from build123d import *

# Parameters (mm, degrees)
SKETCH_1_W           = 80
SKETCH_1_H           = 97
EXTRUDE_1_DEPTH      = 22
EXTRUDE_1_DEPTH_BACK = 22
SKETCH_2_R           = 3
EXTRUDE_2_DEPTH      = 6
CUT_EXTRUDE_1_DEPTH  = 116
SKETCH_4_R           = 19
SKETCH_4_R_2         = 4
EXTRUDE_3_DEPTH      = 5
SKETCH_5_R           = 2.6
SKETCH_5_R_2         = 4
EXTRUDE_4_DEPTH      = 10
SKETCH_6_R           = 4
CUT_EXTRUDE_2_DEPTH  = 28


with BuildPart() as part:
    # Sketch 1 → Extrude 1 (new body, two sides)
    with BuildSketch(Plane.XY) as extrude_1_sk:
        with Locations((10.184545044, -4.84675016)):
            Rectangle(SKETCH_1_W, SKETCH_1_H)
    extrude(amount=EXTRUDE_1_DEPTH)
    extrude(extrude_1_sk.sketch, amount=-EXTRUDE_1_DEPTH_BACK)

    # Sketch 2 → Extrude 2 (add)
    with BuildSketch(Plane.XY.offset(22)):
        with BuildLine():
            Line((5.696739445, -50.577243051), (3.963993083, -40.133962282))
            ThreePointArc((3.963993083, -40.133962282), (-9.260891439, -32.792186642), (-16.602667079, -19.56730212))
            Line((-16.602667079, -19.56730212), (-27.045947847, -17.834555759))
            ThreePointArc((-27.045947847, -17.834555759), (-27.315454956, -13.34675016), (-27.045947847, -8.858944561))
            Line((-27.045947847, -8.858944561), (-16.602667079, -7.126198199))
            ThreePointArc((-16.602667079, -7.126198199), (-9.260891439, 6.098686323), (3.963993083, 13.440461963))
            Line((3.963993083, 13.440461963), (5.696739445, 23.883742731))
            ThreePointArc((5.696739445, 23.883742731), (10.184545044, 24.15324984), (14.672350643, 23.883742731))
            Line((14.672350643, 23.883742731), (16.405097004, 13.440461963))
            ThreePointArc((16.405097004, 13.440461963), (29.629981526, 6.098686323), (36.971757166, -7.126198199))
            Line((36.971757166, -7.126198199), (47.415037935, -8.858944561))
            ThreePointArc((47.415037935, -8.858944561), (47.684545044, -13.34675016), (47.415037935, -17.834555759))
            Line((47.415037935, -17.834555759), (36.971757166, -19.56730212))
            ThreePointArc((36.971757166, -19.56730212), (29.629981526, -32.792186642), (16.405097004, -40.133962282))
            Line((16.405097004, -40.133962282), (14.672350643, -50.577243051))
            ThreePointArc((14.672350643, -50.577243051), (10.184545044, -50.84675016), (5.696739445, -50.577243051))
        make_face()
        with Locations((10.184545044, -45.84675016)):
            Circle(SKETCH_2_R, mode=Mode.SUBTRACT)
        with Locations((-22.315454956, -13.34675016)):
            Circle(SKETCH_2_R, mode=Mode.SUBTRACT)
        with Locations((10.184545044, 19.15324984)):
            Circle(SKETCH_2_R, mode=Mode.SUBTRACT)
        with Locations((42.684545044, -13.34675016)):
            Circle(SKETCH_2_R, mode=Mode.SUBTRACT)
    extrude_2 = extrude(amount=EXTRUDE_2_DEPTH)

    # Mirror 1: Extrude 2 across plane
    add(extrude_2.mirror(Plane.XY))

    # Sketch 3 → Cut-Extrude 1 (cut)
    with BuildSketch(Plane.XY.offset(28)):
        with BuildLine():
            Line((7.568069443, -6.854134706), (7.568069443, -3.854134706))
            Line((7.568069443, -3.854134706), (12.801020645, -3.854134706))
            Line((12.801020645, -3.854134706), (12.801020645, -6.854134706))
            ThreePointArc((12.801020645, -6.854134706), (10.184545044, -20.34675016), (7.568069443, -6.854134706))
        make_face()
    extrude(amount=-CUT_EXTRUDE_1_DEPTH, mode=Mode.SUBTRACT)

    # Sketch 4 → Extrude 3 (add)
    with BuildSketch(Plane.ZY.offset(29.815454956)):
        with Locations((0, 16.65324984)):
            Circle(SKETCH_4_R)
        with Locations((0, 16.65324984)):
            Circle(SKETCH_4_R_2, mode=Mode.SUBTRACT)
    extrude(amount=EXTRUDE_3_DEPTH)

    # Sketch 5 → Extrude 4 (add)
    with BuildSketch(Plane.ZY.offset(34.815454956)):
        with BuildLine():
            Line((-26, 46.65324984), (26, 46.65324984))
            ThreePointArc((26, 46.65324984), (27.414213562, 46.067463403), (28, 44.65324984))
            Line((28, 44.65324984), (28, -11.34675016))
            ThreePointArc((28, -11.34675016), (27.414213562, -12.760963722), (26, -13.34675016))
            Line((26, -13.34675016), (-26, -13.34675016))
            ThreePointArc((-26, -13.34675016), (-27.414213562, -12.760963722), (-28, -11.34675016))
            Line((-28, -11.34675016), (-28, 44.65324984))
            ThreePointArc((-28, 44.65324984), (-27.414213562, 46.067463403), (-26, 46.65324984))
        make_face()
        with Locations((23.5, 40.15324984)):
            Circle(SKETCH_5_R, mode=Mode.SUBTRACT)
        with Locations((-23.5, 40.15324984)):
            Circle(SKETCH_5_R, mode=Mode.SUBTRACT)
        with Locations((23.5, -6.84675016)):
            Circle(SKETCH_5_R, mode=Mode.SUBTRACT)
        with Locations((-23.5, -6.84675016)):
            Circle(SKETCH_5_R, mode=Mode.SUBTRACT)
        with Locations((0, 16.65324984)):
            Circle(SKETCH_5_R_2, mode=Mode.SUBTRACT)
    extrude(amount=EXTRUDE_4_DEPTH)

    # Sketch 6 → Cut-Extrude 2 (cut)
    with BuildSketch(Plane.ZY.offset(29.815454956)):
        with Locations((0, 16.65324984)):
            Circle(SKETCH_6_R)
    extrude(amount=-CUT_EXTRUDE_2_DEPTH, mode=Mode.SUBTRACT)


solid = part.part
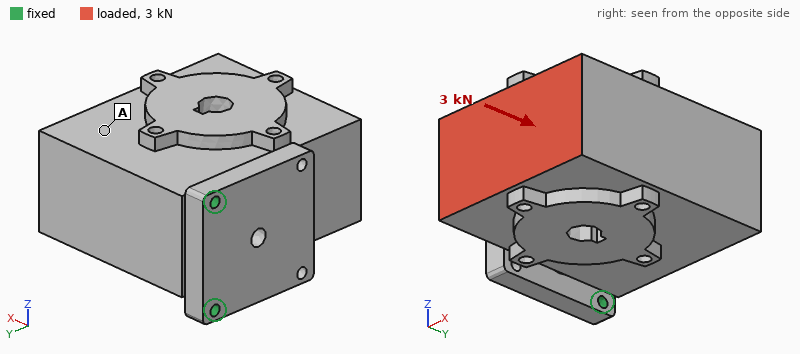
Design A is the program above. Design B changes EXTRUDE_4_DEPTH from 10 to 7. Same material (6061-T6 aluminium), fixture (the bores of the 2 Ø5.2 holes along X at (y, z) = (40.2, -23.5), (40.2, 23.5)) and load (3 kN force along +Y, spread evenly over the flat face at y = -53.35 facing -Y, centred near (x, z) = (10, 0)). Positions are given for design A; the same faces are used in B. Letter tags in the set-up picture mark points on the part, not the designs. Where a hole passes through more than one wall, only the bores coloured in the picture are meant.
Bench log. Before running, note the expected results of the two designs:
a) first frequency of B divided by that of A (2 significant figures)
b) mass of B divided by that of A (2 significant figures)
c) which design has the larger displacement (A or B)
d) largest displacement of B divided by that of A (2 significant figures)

0.66
0.98
B
2.3
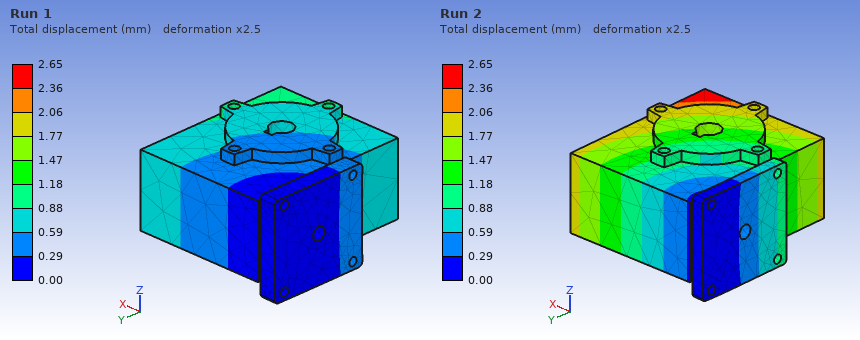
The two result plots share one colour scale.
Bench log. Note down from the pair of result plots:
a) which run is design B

Run 2
